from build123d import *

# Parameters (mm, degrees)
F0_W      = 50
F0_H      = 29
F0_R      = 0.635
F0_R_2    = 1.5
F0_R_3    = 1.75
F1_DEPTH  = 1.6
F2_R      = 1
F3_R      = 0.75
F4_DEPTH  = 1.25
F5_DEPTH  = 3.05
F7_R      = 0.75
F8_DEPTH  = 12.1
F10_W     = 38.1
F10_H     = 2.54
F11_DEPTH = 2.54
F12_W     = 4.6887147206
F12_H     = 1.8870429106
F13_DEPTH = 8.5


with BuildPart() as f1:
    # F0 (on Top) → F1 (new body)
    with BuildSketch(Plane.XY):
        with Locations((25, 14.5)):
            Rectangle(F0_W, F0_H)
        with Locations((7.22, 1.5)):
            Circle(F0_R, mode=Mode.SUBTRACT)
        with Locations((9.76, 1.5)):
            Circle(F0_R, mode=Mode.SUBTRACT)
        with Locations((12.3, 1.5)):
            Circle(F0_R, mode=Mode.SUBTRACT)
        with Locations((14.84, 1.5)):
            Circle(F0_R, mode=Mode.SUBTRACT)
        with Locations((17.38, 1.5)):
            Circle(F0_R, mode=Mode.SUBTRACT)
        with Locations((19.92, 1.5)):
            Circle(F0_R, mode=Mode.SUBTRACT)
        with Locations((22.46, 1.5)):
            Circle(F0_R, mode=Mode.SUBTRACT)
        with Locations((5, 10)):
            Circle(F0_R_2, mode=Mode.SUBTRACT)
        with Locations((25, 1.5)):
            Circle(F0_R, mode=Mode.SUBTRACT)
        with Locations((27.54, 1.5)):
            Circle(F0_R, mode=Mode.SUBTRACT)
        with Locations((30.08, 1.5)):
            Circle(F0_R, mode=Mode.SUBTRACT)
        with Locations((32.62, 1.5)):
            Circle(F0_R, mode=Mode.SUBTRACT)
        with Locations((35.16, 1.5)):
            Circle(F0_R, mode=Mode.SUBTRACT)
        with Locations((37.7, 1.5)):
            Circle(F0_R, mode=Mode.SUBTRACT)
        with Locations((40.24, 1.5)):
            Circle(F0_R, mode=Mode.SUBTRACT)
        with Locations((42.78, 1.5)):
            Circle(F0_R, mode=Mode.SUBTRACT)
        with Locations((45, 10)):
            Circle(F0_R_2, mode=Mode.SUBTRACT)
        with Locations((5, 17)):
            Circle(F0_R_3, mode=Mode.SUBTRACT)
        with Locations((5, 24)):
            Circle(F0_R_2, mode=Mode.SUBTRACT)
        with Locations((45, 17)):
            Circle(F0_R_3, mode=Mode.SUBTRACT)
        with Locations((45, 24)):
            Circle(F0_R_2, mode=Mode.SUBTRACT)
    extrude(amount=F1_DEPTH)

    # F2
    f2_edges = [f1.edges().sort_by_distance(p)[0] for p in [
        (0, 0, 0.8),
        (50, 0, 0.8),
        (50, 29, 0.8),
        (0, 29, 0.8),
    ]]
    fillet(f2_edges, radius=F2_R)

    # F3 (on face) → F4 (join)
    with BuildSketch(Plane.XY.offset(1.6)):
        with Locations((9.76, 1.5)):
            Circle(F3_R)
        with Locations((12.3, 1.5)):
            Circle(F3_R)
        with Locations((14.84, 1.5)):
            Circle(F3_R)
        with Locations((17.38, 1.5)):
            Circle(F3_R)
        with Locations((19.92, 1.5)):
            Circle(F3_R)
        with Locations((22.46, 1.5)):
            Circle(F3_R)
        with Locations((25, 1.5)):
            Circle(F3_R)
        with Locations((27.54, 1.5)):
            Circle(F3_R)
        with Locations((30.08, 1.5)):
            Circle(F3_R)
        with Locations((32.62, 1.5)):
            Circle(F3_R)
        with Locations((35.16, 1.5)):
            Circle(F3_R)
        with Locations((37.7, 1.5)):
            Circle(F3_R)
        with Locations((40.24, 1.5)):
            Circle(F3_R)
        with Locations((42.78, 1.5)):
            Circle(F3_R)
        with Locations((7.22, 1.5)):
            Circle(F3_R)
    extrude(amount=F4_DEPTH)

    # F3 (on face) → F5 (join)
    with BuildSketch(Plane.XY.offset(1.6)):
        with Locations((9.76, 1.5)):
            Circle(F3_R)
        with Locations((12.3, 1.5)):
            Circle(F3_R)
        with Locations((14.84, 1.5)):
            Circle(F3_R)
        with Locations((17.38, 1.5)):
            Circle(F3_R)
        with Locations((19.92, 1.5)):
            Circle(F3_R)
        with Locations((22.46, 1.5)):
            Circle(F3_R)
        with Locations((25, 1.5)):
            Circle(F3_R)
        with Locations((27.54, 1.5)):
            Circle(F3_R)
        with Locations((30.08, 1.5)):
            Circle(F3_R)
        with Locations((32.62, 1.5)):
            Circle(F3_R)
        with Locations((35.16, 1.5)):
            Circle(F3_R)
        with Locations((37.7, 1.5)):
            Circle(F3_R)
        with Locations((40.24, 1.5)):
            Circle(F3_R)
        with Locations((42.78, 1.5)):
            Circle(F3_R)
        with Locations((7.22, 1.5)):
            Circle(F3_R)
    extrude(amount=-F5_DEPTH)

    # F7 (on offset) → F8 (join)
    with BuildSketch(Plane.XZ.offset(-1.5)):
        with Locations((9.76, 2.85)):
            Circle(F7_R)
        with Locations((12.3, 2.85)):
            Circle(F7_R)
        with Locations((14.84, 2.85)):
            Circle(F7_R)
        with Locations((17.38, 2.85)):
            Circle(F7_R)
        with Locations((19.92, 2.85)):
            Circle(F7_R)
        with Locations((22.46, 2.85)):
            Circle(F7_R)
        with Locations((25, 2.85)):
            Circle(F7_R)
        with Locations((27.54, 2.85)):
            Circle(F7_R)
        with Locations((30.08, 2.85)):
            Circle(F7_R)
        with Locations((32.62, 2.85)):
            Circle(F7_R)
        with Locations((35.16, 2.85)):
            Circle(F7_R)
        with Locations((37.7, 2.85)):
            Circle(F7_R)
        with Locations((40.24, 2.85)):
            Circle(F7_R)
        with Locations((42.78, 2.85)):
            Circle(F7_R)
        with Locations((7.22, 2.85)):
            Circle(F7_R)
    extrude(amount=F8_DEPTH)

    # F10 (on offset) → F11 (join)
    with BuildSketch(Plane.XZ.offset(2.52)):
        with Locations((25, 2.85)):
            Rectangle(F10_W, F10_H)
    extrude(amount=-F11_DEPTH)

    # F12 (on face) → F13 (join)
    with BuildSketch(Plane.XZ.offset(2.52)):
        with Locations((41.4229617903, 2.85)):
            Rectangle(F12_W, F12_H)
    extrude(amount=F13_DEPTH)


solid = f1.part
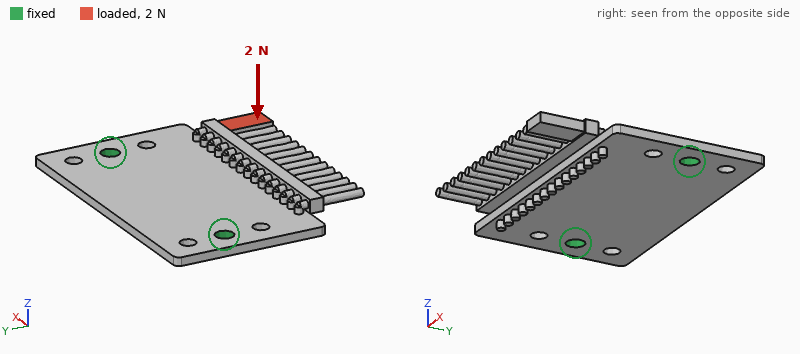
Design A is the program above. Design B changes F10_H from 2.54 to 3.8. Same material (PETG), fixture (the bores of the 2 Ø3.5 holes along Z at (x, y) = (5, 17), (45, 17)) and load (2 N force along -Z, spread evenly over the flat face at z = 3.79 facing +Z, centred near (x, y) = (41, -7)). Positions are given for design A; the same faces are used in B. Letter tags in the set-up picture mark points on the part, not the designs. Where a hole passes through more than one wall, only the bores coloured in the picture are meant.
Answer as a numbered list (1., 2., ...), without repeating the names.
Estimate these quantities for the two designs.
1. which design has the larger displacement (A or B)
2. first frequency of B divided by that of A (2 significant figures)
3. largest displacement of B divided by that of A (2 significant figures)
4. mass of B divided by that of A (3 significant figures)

1. A
2. 0.96
3. 0.89
4. 1.04
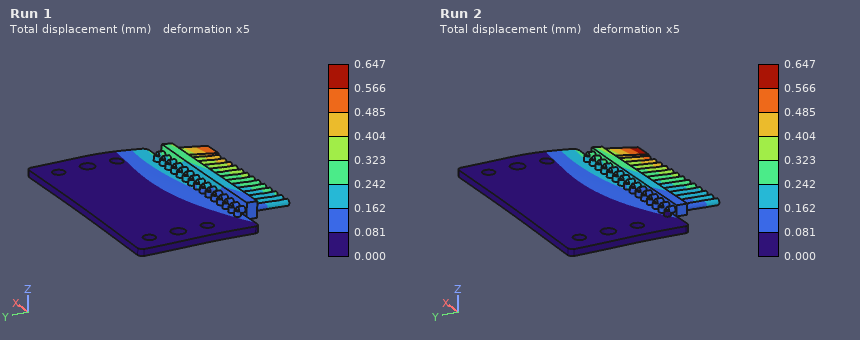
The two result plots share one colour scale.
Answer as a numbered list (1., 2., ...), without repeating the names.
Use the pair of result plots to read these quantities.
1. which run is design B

1. Run 1
